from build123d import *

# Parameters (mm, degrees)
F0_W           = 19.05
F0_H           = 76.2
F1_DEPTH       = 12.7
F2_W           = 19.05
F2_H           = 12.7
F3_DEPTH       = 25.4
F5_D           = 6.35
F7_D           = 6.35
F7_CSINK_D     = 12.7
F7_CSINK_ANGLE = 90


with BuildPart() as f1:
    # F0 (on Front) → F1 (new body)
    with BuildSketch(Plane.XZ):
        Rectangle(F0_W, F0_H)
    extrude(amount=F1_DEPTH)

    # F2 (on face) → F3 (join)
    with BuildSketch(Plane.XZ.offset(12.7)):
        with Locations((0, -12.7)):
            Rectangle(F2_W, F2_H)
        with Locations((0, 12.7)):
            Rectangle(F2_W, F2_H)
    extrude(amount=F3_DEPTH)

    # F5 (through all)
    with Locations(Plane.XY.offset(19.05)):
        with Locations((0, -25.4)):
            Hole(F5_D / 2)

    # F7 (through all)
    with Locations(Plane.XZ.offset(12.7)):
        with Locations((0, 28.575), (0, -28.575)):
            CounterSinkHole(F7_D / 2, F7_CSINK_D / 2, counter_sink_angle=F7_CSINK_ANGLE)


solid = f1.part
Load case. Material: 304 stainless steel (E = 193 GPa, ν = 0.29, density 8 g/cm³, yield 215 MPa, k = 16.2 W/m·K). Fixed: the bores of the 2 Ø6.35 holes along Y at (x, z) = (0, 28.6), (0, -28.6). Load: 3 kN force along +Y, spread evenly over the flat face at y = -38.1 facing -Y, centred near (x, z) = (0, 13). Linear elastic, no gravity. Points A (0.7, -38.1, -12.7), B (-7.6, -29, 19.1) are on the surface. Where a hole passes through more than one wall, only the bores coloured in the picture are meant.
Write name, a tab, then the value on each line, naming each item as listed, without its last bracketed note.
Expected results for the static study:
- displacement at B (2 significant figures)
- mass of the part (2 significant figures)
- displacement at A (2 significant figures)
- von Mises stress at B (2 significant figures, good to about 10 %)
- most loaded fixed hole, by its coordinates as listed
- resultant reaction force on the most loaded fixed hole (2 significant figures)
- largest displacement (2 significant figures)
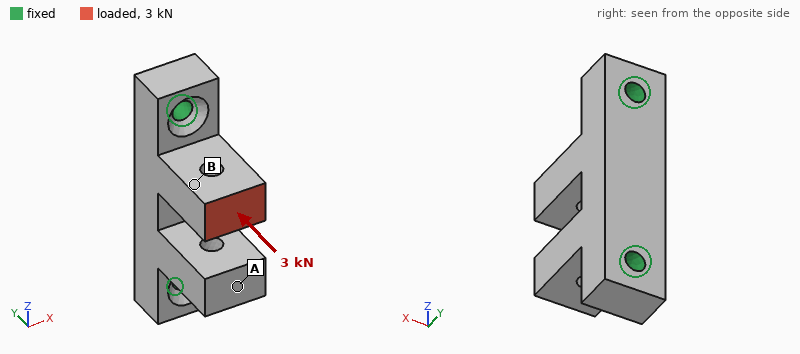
displacement at B	5.7 µm
mass of the part	230 g
displacement at A	6.1 µm
von Mises stress at B	16 MPa
most loaded fixed hole, by its coordinates as listed	(0, 28.6)
resultant reaction force on the most loaded fixed hole	2.4 kN
largest displacement	9.2 µm
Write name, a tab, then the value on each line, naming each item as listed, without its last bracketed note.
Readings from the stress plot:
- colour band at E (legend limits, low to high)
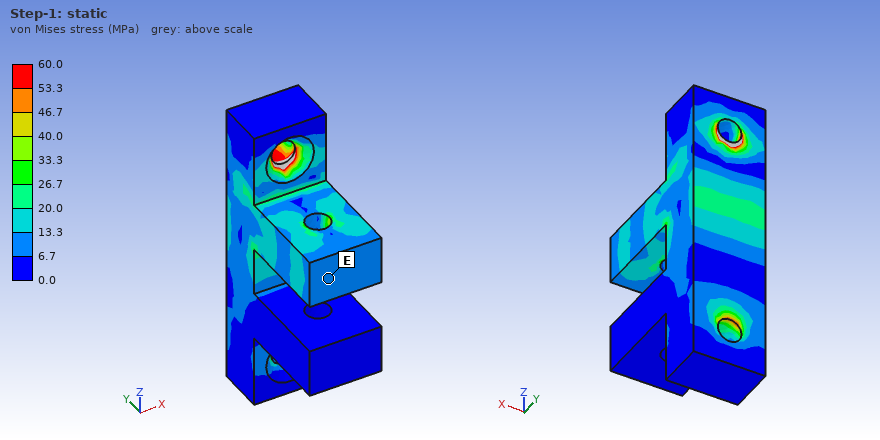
colour band at E	6.7 to 13.3 MPa
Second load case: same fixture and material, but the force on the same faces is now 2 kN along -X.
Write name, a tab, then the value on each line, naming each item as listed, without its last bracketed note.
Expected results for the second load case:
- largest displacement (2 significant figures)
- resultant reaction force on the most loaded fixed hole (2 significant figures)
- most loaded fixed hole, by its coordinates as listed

largest displacement	56 µm
resultant reaction force on the most loaded fixed hole	1.6 kN
most loaded fixed hole, by its coordinates as listed	(0, 28.6)
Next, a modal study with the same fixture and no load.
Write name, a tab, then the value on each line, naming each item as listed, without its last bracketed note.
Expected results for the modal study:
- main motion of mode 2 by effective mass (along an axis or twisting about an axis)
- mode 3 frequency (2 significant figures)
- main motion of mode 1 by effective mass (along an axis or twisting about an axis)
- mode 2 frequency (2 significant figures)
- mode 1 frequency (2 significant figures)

main motion of mode 2 by effective mass	along Y
mode 3 frequency	8700 Hz
main motion of mode 1 by effective mass	along X
mode 2 frequency	7100 Hz
mode 1 frequency	5700 Hz
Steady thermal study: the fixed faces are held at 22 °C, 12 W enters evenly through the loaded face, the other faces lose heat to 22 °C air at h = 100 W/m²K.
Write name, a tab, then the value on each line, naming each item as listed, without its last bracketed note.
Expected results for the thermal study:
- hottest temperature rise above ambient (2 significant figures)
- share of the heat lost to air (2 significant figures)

hottest temperature rise above ambient	72 K
share of the heat lost to air	72 %
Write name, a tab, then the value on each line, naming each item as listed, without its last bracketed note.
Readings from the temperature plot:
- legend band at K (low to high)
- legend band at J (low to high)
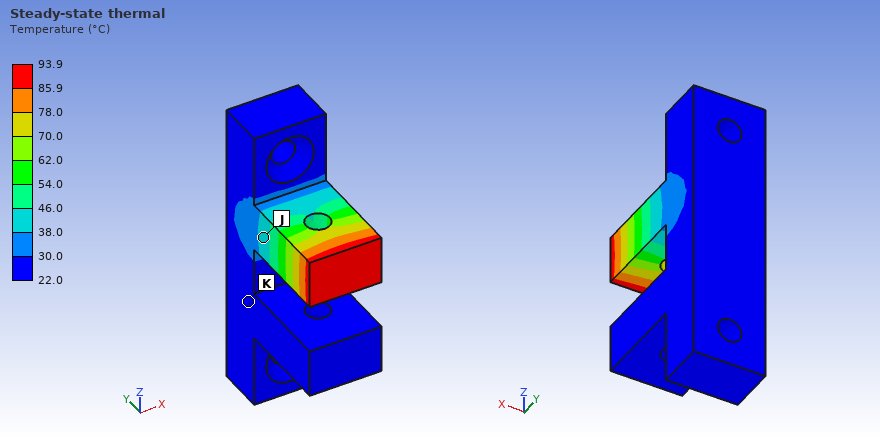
legend band at K	22.0 to 30.0 °C
legend band at J	38.0 to 46.0 °C
